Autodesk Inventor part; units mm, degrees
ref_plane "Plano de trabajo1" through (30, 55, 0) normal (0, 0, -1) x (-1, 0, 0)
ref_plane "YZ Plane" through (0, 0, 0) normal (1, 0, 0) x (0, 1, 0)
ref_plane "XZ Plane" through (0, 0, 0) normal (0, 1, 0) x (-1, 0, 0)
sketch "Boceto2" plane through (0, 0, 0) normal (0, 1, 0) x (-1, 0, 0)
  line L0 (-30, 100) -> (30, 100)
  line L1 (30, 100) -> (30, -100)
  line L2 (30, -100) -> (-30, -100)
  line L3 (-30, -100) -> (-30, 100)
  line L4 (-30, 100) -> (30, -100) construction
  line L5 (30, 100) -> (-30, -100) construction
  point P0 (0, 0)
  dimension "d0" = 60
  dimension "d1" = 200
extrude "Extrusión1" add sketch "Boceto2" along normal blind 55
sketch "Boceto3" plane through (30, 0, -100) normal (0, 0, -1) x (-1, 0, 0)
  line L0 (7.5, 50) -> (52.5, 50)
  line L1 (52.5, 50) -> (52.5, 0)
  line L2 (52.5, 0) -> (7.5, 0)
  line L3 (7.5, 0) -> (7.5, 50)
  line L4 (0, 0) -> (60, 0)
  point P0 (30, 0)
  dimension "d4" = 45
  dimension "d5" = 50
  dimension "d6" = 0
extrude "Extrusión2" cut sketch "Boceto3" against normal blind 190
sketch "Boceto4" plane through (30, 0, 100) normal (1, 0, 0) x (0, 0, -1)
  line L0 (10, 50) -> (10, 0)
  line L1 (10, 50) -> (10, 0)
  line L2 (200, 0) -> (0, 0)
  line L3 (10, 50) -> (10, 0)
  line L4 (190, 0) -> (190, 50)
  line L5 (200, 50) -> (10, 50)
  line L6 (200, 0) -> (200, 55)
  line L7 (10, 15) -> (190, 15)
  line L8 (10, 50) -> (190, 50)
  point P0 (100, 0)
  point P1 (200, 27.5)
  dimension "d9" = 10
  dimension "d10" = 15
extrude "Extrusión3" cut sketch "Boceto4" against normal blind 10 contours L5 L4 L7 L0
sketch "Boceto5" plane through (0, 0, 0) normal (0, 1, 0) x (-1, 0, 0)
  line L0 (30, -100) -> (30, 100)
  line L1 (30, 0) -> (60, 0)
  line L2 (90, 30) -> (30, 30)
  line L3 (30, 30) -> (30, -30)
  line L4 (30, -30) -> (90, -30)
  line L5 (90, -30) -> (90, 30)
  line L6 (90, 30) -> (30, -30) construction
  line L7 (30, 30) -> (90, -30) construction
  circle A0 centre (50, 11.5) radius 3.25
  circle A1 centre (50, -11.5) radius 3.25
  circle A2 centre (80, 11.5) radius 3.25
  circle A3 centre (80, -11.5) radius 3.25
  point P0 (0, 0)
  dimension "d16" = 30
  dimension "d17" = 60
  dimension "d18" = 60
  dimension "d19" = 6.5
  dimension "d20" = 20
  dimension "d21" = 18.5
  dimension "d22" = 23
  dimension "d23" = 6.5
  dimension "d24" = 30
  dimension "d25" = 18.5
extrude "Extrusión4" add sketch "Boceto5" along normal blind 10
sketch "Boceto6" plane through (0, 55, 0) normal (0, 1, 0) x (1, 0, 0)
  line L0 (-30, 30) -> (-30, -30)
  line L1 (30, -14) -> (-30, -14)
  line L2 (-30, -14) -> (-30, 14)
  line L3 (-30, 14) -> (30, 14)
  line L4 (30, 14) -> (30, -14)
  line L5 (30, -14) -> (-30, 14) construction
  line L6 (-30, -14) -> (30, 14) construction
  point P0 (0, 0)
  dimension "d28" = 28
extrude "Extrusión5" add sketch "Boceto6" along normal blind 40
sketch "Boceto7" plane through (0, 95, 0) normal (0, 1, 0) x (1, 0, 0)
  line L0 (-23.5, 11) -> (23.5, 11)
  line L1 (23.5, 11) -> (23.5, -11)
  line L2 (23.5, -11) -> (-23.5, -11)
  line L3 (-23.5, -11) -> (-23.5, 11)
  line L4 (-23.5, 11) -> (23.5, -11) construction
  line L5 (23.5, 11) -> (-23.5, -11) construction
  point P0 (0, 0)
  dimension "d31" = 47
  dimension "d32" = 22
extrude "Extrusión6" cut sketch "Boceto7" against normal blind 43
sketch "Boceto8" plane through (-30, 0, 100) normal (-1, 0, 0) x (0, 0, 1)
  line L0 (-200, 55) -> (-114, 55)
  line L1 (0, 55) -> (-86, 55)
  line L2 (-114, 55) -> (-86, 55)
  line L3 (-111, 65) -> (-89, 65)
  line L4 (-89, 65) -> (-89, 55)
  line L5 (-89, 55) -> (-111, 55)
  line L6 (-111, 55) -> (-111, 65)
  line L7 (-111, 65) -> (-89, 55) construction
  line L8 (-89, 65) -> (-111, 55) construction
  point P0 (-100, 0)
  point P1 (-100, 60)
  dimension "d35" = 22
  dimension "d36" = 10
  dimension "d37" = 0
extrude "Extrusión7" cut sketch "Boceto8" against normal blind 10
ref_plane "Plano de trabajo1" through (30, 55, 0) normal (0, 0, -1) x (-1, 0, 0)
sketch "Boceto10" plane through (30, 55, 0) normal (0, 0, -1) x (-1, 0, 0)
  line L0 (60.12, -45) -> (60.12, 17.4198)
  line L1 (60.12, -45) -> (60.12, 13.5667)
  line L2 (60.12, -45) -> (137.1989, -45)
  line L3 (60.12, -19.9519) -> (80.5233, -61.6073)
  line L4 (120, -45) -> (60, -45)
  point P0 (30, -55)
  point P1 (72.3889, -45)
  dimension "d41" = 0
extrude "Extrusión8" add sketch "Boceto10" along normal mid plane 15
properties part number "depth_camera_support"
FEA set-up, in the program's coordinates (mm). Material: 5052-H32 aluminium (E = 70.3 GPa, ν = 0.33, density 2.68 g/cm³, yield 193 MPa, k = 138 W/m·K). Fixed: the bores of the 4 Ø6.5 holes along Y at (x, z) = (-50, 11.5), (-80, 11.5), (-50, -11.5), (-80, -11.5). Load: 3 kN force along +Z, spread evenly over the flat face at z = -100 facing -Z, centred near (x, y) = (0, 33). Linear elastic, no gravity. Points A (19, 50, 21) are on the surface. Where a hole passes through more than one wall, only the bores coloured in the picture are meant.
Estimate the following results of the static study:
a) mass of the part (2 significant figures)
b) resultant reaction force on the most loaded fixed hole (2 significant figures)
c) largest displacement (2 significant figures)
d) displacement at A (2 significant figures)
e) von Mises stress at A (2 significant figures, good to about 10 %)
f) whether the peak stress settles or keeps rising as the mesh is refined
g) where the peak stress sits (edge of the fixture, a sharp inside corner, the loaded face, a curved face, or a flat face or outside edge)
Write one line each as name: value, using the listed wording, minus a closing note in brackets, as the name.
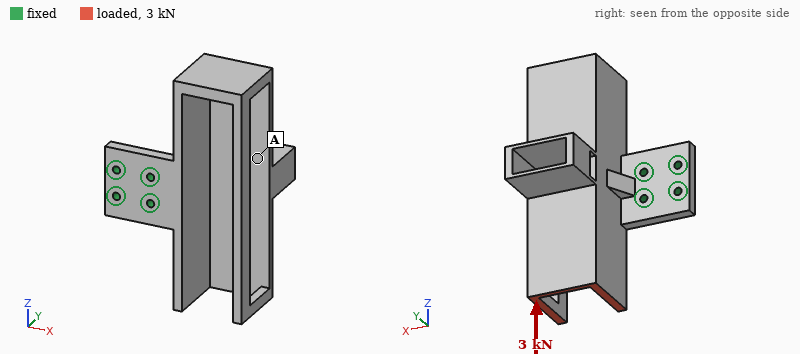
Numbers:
mass of the part: 650 g
resultant reaction force on the most loaded fixed hole: 4.6 kN
largest displacement: 0.64 mm
displacement at A: 0.31 mm
von Mises stress at A: 9.8 MPa
whether the peak stress settles or keeps rising as the mesh is refined: keeps rising
where the peak stress sits: edge of the fixture
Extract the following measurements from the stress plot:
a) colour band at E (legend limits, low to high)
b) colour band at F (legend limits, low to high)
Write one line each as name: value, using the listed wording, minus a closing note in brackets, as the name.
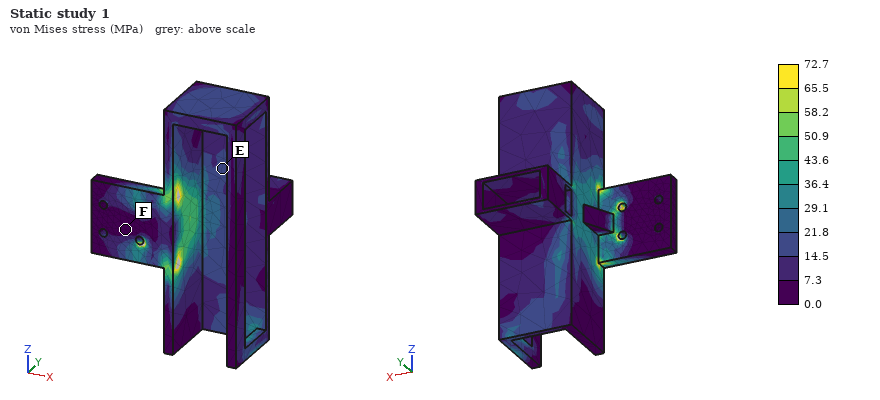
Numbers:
colour band at E: 14.5 to 21.8 MPa
colour band at F: 0.0 to 7.3 MPa
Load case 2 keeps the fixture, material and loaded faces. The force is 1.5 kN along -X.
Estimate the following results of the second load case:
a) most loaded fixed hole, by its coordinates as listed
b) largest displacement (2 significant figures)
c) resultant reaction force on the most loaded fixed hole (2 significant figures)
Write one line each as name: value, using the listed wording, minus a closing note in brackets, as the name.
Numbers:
most loaded fixed hole, by its coordinates as listed: (-50, -11.5)
largest displacement: 2.0 mm
resultant reaction force on the most loaded fixed hole: 3.7 kN
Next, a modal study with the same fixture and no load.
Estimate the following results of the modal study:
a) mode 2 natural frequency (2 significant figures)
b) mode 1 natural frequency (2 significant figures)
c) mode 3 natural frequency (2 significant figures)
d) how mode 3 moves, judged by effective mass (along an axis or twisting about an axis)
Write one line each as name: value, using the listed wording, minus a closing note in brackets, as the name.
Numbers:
mode 2 natural frequency: 400 Hz
mode 1 natural frequency: 330 Hz
mode 3 natural frequency: 560 Hz
how mode 3 moves, judged by effective mass: along X
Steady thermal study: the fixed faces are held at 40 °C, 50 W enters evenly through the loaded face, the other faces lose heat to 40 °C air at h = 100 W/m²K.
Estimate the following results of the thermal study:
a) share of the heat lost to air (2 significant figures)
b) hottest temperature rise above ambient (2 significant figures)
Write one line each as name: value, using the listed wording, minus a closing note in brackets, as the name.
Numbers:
share of the heat lost to air: 87 %
hottest temperature rise above ambient: 36 K
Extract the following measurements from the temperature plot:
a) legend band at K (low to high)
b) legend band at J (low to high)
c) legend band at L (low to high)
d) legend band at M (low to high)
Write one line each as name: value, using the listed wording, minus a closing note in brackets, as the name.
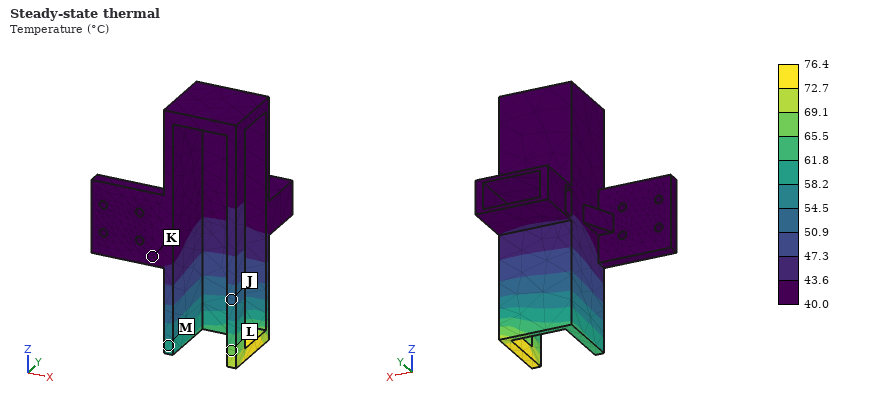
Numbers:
legend band at K: 40.0 to 43.6 °C
legend band at J: 50.9 to 54.5 °C
legend band at L: 65.5 to 69.1 °C
legend band at M: 58.2 to 61.8 °C
